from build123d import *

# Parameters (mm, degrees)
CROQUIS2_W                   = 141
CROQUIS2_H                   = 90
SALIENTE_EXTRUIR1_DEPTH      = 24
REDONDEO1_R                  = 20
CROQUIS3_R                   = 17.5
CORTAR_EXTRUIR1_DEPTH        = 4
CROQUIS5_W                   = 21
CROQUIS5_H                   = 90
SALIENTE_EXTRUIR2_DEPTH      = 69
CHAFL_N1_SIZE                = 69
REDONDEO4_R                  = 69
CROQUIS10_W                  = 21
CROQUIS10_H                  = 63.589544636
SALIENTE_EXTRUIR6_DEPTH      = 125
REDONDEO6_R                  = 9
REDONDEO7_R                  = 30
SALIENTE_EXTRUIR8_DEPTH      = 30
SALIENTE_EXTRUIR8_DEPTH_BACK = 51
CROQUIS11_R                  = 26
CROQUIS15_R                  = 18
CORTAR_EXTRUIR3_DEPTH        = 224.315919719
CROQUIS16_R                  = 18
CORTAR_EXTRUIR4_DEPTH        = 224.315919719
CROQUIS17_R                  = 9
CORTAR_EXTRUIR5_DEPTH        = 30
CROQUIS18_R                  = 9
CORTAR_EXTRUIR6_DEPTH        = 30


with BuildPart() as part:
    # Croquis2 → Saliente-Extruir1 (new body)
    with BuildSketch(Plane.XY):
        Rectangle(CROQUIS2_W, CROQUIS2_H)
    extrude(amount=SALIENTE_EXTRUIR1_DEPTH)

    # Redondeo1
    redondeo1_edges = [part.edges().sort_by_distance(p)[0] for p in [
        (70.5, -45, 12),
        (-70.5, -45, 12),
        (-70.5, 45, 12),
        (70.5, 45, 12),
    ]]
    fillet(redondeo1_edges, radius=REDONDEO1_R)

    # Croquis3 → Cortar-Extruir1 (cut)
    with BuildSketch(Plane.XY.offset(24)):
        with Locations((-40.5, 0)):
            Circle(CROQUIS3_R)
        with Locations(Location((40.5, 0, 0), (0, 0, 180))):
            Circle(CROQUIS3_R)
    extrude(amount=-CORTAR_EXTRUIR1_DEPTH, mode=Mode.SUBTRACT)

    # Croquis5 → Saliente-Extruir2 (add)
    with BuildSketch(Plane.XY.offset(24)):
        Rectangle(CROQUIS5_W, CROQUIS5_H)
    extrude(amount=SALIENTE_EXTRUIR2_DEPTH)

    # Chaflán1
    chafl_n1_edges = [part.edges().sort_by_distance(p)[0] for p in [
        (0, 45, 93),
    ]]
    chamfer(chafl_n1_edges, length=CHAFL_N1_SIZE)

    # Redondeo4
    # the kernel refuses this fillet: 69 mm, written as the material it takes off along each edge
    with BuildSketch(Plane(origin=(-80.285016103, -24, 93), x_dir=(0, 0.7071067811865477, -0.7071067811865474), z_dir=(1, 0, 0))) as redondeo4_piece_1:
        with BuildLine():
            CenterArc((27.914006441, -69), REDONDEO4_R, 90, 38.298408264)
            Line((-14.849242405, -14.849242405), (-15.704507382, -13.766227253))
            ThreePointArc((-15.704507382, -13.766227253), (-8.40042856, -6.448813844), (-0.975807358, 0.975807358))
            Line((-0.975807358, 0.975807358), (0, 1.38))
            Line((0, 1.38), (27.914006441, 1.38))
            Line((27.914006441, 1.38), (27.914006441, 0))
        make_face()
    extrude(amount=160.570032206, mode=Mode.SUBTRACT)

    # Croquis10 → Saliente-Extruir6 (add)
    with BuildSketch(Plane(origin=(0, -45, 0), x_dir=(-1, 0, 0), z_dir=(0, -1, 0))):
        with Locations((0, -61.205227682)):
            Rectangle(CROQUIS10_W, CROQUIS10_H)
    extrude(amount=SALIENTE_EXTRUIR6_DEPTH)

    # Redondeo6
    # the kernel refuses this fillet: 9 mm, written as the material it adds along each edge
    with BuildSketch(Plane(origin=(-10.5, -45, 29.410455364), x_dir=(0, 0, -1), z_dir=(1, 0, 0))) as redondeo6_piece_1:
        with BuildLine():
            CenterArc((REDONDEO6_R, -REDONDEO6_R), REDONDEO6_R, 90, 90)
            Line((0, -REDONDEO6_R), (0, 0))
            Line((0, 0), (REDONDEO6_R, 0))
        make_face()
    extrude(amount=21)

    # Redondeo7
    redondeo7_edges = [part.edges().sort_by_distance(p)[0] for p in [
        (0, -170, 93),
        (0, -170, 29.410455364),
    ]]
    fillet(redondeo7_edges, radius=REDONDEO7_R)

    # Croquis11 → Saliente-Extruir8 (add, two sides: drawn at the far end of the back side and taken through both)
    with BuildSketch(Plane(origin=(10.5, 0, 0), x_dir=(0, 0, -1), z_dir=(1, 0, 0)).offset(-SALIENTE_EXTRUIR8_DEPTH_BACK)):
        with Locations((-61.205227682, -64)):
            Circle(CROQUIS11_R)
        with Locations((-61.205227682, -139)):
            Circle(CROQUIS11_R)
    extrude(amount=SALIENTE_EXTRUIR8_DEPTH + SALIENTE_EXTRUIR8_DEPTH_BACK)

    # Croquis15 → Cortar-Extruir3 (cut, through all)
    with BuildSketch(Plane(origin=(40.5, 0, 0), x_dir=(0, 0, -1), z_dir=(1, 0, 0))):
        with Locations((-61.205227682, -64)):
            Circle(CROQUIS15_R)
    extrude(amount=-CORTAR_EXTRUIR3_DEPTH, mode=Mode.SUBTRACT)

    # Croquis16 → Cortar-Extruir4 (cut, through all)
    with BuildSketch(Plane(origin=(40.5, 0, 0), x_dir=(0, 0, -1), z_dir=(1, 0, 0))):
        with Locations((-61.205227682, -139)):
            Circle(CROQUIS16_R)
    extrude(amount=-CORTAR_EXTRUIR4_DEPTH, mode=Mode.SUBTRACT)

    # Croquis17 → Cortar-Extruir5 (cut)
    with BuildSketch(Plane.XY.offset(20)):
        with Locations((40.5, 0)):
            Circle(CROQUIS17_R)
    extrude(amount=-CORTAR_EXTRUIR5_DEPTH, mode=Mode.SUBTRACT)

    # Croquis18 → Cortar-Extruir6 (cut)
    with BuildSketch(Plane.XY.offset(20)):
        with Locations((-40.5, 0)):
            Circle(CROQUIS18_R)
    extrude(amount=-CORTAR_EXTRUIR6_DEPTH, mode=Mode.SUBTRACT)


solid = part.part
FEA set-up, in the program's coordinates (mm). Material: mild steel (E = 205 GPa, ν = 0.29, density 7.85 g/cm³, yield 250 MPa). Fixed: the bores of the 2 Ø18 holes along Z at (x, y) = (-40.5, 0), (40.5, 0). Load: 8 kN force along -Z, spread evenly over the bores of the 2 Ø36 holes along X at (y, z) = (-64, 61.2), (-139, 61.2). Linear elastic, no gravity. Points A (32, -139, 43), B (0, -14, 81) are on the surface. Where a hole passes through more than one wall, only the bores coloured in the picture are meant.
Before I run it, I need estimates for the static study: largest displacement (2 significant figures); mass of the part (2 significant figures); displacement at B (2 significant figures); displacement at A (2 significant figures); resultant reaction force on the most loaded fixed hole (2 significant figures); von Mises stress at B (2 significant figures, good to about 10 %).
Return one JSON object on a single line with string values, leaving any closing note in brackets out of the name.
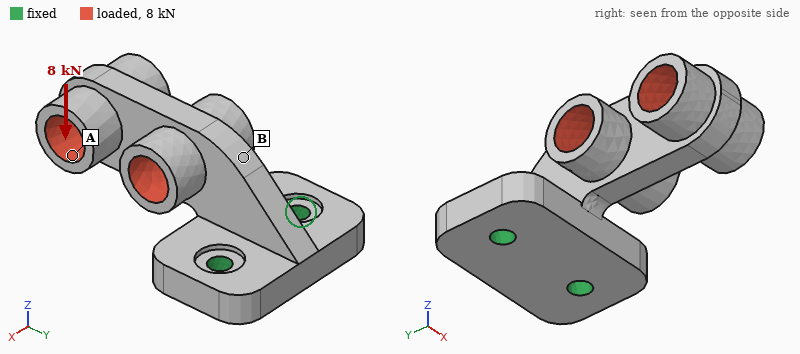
{"largest displacement": "0.18 mm", "mass of the part": "4.8 kg", "displacement at B": "0.050 mm", "displacement at A": "0.14 mm", "resultant reaction force on the most loaded fixed hole": "4.7 kN", "von Mises stress at B": "28 MPa"}
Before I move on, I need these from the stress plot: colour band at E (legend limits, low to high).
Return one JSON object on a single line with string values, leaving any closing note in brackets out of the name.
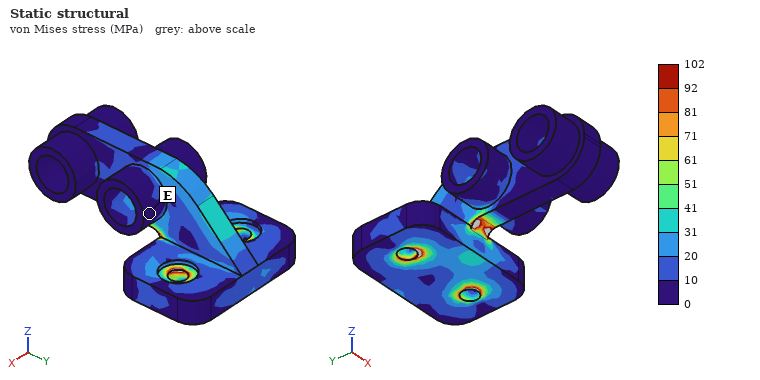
{"colour band at E": "0 to 10 MPa"}
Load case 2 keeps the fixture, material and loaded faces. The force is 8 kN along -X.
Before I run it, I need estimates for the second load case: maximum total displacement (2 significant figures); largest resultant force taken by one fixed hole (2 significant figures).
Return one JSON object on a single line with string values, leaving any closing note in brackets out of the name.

{"maximum total displacement": "0.46 mm", "largest resultant force taken by one fixed hole": "11 kN"}
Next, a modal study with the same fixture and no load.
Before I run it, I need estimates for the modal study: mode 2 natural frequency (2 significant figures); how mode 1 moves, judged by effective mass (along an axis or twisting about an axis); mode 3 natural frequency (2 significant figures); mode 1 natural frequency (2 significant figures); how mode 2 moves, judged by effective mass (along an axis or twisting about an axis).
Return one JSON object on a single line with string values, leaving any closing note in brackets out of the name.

{"mode 2 natural frequency": "860 Hz", "how mode 1 moves, judged by effective mass": "along X", "mode 3 natural frequency": "1500 Hz", "mode 1 natural frequency": "570 Hz", "how mode 2 moves, judged by effective mass": "along Z"}
